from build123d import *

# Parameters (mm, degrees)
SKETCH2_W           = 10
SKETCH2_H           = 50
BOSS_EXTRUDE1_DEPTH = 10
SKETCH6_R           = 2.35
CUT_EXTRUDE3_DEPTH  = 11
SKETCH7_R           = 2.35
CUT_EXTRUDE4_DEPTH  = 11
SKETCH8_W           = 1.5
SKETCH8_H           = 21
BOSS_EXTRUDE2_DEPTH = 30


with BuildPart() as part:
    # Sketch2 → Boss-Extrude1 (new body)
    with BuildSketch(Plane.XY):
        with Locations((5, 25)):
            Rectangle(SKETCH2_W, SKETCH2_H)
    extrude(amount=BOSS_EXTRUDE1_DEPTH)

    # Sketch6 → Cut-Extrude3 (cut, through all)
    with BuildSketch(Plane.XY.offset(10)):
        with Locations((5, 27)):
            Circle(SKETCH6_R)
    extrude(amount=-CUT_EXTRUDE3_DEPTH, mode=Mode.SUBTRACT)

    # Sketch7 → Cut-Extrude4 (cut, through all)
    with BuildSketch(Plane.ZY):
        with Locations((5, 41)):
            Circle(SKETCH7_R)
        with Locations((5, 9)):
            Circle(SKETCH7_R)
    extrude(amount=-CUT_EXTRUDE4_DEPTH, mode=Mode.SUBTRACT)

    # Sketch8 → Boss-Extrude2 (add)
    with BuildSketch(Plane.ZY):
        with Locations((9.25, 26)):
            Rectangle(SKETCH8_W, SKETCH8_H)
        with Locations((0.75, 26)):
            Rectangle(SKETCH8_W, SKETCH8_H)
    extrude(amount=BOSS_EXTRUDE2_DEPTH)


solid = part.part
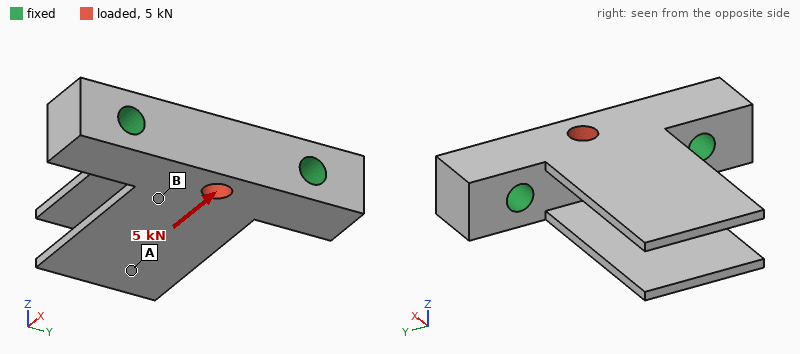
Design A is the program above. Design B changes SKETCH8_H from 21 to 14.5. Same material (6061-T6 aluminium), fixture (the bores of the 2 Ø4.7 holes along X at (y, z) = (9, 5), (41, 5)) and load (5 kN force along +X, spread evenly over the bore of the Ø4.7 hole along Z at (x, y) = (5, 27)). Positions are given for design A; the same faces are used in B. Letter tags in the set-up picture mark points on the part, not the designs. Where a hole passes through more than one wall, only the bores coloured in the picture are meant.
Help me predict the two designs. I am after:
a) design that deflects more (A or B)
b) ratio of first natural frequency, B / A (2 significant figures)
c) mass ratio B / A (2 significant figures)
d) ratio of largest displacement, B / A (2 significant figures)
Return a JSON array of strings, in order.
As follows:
["B", "0.99", "0.91", "1.1"]
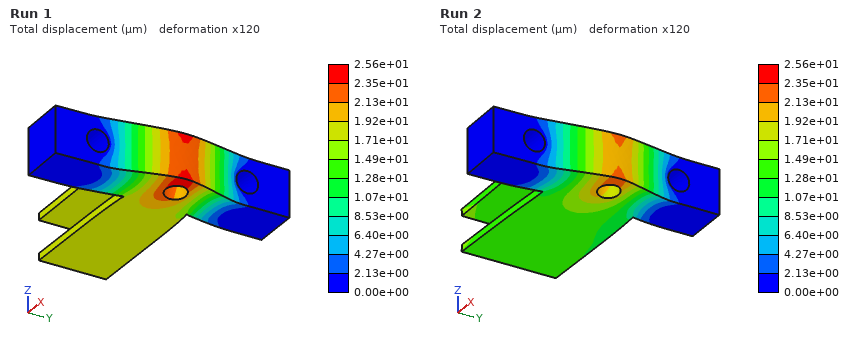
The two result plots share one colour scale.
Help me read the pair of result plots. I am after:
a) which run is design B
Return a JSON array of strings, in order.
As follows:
["Run 1"]
